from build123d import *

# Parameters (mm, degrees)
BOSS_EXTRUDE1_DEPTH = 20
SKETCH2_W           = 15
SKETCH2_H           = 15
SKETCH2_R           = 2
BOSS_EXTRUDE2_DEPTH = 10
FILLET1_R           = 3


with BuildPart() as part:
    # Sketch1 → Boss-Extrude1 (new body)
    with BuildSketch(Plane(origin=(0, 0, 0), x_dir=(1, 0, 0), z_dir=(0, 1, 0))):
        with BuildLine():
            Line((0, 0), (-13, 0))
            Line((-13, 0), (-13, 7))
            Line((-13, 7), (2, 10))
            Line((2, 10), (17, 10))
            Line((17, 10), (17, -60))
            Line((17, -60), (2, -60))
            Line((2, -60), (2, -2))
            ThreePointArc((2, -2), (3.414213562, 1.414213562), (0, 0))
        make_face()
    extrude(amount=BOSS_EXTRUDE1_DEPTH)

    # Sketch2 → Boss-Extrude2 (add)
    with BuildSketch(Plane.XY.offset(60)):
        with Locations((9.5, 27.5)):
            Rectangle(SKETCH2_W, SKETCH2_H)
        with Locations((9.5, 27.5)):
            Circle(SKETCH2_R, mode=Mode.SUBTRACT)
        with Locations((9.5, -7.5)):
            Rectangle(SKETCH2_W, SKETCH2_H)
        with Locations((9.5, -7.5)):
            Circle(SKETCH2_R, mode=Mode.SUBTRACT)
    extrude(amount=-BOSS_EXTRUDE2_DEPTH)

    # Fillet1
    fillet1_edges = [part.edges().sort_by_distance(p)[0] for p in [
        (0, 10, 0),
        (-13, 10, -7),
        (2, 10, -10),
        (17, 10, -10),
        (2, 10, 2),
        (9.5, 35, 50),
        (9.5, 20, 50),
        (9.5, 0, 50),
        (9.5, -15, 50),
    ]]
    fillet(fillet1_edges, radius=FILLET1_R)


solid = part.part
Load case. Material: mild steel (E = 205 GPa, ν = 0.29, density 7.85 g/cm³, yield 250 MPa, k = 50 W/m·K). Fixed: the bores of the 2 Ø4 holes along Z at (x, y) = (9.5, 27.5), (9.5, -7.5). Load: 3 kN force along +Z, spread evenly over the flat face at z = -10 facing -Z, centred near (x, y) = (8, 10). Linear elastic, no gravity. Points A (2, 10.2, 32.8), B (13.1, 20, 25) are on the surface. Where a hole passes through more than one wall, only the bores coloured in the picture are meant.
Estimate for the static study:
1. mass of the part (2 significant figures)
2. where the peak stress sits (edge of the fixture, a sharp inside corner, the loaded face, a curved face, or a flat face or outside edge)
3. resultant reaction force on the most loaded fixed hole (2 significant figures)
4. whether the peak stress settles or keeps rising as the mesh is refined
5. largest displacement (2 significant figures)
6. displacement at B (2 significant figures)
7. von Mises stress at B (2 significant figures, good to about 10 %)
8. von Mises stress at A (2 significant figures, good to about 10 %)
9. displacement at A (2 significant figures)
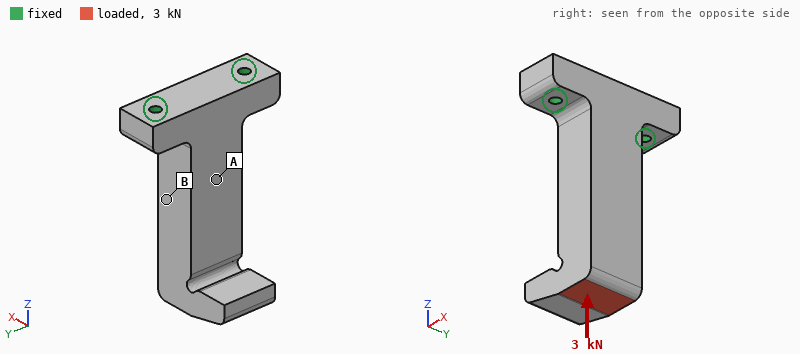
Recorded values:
220 g
edge of the fixture
1.6 kN
keeps rising
16 µm
4.5 µm
7.3 MPa
16 MPa
4.7 µm
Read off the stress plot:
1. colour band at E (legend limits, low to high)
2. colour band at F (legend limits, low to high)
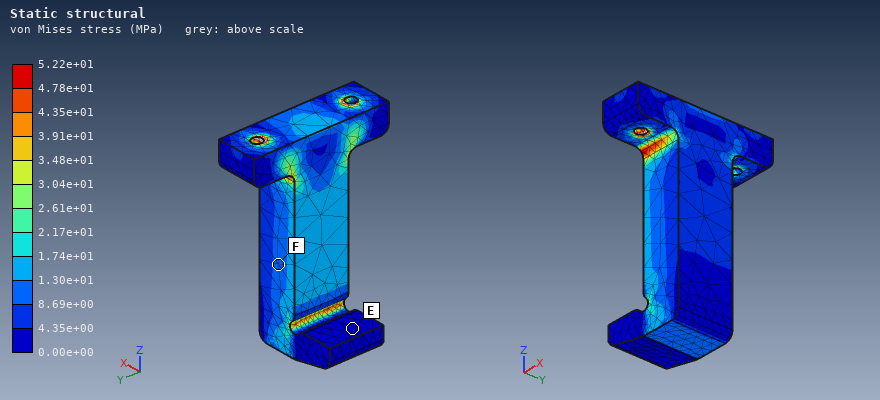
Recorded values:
0.00e+00 to 4.35e+00 MPa
8.69e+00 to 1.30e+01 MPa
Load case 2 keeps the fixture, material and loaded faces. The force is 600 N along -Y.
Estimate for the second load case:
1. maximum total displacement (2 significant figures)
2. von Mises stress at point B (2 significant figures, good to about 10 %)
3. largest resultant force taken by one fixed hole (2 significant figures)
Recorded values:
32 µm
21 MPa
1.4 kN
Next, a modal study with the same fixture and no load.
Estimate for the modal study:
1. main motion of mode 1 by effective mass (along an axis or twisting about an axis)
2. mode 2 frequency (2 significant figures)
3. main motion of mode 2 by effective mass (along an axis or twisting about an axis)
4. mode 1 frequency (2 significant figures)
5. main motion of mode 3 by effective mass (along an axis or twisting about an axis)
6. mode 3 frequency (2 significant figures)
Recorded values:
along X
3000 Hz
along Y
1600 Hz
twisting about Z
7600 Hz
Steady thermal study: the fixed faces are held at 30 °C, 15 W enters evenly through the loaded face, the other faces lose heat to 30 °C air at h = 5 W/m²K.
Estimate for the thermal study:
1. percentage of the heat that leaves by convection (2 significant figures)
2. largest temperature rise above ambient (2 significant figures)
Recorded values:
7.7 %
70 K
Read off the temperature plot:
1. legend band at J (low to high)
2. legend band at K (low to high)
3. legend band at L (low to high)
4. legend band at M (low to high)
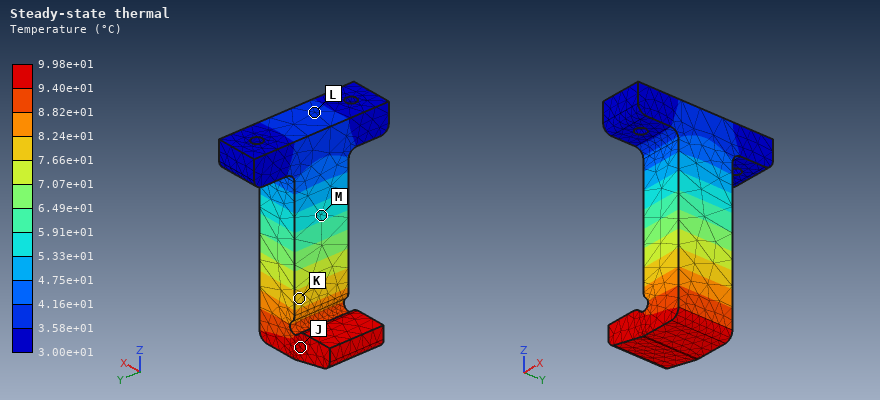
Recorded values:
9.40e+01 to 9.98e+01 °C
7.66e+01 to 8.24e+01 °C
3.58e+01 to 4.16e+01 °C
5.33e+01 to 5.91e+01 °C
